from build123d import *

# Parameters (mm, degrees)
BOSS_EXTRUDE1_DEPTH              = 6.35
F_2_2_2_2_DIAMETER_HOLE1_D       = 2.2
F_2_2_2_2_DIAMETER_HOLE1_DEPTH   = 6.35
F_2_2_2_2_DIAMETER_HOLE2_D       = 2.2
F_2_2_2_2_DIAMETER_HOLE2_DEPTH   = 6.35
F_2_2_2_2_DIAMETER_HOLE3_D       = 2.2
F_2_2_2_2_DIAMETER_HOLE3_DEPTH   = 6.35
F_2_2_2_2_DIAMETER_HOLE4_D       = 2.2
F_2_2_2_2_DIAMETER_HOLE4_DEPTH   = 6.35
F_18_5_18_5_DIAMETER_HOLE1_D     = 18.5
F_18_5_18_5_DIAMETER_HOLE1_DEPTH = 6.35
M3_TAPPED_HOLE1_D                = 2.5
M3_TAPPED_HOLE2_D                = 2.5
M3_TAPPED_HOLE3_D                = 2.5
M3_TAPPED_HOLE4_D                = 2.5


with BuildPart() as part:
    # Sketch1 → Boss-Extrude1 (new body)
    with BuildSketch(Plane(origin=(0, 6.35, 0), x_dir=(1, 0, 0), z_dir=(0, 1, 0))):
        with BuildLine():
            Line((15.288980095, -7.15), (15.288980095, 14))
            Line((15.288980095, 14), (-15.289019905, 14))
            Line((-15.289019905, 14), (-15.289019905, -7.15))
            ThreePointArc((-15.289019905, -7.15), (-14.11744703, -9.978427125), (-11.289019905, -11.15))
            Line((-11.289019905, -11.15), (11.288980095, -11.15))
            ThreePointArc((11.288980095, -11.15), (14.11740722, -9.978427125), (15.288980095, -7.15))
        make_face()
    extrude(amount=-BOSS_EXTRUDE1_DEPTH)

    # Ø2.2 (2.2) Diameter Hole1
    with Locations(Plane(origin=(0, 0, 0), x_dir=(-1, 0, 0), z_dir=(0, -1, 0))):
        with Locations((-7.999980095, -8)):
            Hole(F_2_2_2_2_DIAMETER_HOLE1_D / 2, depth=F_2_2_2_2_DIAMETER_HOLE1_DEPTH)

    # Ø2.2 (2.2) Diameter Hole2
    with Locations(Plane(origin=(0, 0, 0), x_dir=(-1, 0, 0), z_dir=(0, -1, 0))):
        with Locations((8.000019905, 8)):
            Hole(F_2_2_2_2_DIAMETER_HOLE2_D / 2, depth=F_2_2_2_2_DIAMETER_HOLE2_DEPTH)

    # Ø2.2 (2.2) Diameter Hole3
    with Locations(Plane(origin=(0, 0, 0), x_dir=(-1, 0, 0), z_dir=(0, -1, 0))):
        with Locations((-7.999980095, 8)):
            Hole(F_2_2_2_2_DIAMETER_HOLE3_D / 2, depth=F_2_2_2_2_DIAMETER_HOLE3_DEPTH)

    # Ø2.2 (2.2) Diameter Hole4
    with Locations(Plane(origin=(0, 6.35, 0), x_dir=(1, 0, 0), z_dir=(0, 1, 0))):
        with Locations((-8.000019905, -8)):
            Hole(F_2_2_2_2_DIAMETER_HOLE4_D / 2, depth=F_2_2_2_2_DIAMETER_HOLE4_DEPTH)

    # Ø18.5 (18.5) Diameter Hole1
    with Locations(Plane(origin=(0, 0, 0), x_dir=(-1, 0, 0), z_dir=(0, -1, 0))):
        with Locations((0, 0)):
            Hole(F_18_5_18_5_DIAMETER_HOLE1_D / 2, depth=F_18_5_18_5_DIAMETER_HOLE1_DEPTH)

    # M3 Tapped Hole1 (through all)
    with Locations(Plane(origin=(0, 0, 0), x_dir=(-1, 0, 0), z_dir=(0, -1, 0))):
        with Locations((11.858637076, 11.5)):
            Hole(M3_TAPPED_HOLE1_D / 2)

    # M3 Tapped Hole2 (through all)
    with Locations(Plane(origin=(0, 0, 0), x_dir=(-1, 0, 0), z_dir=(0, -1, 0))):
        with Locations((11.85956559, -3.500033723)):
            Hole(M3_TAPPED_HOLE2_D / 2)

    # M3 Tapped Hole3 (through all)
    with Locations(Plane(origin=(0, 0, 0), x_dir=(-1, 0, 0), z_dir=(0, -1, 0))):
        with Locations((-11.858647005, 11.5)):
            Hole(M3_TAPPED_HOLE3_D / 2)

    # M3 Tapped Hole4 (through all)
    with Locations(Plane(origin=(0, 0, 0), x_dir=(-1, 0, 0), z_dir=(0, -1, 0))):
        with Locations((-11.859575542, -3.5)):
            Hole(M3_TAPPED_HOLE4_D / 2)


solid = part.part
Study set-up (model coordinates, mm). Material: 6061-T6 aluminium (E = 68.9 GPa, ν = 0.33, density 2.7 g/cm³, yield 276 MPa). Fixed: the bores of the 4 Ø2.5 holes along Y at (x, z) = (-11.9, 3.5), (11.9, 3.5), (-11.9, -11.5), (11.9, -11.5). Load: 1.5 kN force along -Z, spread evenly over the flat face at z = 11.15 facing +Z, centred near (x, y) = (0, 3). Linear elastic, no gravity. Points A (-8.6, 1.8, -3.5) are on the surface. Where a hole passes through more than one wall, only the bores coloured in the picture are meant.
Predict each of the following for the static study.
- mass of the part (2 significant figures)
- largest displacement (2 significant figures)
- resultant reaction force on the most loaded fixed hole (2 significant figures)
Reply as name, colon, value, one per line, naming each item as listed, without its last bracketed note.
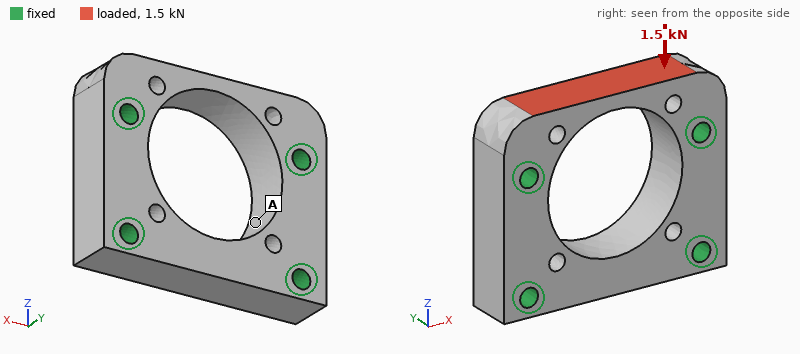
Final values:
mass of the part: 7.9 g
largest displacement: 19 µm
resultant reaction force on the most loaded fixed hole: 870 N
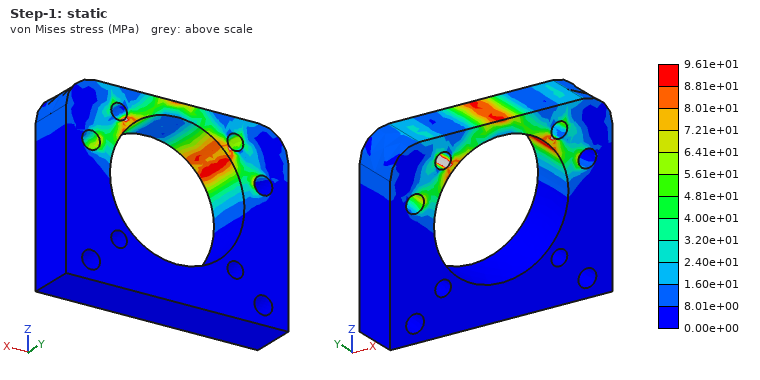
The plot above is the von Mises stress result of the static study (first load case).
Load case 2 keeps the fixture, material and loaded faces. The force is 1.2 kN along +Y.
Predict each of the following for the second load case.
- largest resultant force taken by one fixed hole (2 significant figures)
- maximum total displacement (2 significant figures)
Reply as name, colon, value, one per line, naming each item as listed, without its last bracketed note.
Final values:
largest resultant force taken by one fixed hole: 630 N
maximum total displacement: 37 µm
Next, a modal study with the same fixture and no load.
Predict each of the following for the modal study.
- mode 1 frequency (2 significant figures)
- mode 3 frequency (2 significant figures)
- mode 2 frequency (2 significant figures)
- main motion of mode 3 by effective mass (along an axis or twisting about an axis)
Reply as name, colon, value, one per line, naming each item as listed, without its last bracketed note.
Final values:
mode 1 frequency: 37 kHz
mode 3 frequency: 47 kHz
mode 2 frequency: 44 kHz
main motion of mode 3 by effective mass: along Y
